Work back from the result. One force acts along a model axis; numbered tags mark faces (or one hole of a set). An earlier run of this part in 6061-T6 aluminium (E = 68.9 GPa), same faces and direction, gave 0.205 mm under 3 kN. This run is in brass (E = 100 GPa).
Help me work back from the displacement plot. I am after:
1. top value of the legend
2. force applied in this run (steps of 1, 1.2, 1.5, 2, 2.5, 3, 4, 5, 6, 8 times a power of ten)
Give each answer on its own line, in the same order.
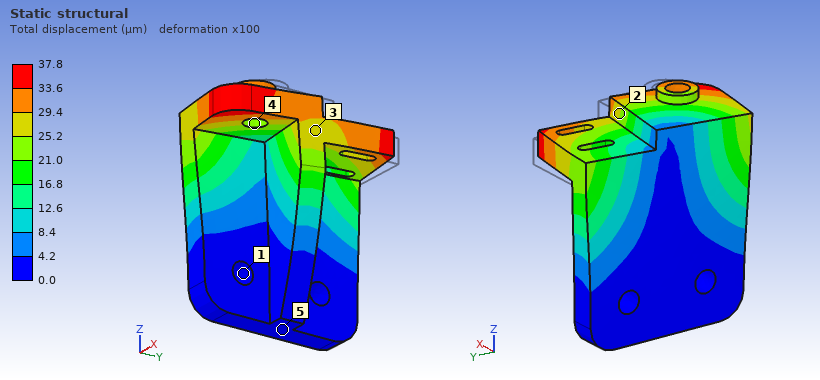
37.8 µm
800 N
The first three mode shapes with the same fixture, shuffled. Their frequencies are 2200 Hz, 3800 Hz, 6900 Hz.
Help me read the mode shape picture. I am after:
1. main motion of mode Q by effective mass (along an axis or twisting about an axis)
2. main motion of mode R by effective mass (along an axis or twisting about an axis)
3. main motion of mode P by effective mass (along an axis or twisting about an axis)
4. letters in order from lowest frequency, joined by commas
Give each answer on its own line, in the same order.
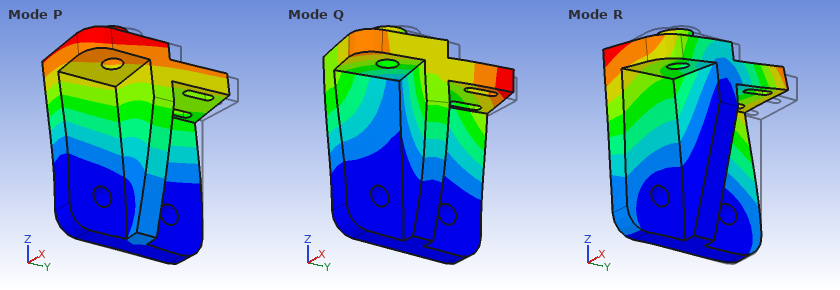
along Y
along Y
along X
P, Q, R
